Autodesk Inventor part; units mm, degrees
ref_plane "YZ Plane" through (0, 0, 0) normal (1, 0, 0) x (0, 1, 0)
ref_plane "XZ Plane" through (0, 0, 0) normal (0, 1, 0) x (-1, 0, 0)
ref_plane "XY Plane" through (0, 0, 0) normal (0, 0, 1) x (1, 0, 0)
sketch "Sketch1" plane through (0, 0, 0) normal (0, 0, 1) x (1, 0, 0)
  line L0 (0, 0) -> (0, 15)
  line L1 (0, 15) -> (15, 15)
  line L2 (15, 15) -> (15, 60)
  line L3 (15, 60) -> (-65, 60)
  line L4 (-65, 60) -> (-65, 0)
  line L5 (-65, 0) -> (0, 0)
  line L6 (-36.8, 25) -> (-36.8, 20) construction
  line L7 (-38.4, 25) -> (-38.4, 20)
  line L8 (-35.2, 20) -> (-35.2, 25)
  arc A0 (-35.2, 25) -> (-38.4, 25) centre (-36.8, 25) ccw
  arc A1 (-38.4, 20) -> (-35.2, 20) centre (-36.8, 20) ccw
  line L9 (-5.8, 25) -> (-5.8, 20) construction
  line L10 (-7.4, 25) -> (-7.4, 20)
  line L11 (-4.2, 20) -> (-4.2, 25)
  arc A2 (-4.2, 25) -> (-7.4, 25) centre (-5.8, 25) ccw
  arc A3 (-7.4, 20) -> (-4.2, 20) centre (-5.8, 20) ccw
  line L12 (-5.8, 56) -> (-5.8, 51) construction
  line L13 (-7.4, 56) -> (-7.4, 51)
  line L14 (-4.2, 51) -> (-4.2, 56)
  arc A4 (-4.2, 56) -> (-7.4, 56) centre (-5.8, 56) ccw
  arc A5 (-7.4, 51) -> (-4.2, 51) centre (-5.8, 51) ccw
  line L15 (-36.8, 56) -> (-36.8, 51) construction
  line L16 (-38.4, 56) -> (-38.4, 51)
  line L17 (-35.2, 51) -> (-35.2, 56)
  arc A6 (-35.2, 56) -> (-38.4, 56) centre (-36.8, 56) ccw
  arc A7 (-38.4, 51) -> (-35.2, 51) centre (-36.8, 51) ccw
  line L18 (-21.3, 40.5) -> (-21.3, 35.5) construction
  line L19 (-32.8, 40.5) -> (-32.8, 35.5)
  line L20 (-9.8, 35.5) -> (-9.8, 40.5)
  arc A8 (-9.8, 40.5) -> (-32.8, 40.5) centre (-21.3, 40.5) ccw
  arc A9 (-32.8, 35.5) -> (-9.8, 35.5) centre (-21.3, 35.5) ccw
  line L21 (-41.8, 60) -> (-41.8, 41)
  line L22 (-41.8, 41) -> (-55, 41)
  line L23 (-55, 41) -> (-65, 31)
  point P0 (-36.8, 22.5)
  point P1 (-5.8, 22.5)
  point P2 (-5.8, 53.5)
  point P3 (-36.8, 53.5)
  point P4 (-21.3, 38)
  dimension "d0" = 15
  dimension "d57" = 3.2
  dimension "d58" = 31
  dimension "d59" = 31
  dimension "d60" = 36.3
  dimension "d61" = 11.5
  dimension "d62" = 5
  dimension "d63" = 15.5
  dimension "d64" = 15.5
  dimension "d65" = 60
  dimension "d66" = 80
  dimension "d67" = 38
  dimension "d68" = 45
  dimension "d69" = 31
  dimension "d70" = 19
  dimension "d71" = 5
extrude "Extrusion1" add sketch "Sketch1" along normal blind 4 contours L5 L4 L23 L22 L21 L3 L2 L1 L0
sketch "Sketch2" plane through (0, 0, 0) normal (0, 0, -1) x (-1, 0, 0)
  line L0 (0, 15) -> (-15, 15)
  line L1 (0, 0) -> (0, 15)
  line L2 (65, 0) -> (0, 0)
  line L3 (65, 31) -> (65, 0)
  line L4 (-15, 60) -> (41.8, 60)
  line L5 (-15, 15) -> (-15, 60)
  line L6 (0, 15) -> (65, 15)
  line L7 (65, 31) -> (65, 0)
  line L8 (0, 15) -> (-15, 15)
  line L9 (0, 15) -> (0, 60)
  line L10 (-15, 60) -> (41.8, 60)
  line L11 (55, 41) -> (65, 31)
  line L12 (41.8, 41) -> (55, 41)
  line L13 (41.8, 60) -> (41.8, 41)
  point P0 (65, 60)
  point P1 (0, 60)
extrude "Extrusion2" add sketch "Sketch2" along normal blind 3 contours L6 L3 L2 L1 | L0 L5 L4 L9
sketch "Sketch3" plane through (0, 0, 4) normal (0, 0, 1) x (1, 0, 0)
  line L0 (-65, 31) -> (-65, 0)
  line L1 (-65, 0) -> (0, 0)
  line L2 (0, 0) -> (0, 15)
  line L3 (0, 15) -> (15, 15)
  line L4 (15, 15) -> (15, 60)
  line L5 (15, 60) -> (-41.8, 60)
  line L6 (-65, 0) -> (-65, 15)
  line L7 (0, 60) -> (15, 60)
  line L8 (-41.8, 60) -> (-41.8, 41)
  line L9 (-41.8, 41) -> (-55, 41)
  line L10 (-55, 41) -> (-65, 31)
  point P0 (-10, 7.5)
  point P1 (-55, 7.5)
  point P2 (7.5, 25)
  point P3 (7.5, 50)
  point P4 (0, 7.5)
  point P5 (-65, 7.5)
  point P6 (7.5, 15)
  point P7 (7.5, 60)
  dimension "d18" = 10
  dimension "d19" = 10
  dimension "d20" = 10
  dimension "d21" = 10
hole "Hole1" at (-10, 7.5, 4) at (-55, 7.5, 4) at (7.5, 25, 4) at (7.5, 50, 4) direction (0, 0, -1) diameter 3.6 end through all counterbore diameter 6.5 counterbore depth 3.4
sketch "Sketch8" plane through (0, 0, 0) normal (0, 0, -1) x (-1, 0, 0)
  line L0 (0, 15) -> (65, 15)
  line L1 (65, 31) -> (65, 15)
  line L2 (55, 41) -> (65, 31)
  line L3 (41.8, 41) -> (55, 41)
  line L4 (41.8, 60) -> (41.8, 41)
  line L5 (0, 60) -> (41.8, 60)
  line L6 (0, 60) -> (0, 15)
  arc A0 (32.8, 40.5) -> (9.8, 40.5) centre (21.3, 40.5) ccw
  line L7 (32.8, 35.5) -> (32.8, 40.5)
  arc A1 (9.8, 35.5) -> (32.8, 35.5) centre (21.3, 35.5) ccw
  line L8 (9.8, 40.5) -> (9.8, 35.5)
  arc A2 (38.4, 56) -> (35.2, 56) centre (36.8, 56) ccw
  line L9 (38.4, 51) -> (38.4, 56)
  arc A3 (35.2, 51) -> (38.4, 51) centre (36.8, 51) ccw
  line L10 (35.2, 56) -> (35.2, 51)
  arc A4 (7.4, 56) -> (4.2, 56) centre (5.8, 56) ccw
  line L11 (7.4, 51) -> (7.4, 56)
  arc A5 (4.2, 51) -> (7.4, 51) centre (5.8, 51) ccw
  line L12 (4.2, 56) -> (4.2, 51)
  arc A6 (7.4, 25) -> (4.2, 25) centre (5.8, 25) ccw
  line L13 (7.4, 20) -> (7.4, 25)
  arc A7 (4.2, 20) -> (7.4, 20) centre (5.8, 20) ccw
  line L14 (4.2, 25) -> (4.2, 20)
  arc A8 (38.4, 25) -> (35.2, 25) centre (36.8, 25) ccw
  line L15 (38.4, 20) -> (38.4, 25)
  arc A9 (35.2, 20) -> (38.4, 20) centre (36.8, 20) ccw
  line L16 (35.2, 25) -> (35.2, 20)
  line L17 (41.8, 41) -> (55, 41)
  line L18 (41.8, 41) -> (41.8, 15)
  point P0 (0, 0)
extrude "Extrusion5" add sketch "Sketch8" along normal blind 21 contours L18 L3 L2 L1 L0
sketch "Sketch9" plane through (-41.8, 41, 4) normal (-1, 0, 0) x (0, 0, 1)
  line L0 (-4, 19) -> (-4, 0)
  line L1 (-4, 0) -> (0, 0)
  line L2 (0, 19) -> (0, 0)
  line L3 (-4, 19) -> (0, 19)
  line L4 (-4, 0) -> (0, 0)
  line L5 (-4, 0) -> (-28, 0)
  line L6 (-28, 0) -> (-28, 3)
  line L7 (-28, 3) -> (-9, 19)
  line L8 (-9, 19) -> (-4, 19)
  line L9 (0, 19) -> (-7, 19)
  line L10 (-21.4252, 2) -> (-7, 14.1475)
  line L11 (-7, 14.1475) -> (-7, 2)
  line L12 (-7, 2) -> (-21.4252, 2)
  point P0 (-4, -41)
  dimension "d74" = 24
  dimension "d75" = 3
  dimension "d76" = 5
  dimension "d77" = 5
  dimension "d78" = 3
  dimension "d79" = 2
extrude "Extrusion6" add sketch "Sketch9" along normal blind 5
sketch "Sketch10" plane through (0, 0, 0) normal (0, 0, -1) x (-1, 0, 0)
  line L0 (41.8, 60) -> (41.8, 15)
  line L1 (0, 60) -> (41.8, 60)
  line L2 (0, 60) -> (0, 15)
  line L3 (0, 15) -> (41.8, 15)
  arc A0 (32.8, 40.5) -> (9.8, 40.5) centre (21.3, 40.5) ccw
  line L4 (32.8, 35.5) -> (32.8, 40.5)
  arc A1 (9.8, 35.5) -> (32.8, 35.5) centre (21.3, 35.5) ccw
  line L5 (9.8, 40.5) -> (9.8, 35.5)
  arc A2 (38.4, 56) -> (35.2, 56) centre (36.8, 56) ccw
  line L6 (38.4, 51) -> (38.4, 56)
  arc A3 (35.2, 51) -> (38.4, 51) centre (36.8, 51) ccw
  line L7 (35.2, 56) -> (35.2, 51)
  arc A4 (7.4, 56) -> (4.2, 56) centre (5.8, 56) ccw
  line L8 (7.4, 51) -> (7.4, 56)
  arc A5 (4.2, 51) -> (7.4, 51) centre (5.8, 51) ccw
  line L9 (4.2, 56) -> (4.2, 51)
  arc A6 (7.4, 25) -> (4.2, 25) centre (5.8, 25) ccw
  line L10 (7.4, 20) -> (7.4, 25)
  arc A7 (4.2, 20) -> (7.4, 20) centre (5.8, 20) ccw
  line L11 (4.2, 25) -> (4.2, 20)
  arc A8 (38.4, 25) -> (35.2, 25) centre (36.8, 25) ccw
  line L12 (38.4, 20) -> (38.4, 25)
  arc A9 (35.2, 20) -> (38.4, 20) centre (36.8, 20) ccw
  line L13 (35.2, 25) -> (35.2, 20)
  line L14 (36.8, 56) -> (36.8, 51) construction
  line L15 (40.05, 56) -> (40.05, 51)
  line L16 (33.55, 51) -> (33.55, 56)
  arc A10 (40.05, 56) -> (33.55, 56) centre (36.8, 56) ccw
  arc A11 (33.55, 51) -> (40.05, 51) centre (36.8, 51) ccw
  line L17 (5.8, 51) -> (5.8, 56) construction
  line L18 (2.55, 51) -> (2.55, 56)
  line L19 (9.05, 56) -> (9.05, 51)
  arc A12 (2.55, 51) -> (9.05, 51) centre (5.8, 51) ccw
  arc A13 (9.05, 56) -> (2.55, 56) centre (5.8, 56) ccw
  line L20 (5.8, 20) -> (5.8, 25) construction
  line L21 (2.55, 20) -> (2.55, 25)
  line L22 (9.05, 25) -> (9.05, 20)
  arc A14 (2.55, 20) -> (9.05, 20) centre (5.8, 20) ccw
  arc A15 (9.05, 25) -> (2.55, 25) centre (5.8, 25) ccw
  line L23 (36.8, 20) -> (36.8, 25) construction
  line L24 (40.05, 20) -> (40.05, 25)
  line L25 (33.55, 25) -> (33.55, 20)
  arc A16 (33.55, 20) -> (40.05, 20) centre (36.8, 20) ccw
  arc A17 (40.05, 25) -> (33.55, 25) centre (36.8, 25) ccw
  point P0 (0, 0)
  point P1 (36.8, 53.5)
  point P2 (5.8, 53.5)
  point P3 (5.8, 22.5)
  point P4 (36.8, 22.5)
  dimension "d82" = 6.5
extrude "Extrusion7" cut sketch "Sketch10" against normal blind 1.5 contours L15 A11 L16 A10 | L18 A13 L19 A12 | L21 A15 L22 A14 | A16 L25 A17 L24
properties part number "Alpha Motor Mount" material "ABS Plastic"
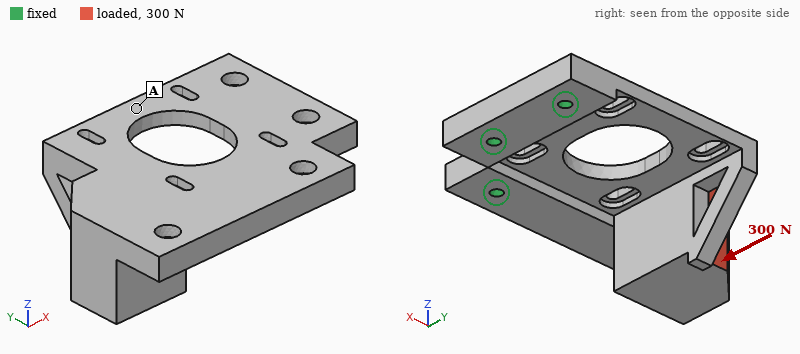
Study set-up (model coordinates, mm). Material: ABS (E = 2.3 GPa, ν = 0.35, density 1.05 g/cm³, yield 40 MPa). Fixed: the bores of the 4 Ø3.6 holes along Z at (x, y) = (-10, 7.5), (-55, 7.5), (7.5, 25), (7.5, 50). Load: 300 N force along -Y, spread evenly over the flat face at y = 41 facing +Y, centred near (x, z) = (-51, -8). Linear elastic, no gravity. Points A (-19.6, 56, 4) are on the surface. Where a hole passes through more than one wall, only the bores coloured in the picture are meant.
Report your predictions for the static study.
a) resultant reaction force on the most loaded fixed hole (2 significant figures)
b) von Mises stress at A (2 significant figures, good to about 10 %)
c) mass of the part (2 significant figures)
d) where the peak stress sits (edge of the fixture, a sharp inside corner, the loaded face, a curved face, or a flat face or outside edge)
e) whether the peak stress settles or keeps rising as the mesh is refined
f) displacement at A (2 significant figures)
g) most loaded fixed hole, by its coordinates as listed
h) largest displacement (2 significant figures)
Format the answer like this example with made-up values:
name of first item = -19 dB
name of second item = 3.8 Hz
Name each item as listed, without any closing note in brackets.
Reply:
resultant reaction force on the most loaded fixed hole = 300 N
von Mises stress at A = 2.4 MPa
mass of the part = 33 g
where the peak stress sits = edge of the fixture
whether the peak stress settles or keeps rising as the mesh is refined = keeps rising
displacement at A = 0.43 mm
most loaded fixed hole, by its coordinates as listed = (-55, 7.5)
largest displacement = 1.1 mm
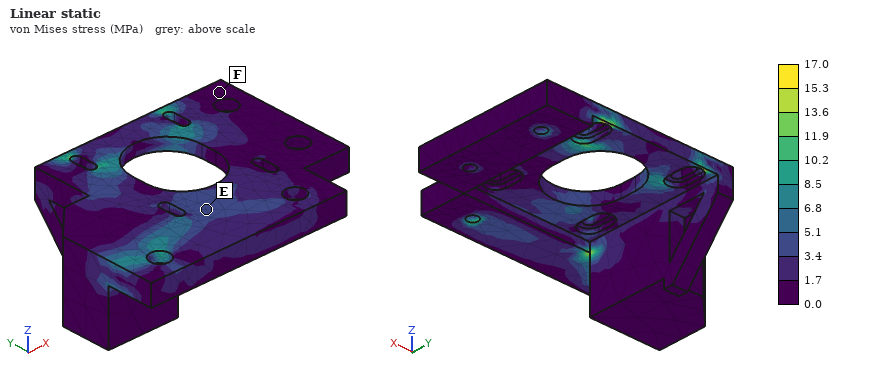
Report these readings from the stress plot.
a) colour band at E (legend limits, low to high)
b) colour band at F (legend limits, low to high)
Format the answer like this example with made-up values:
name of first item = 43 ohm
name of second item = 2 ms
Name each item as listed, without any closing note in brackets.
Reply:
colour band at E = 3.4 to 5.1 MPa
colour band at F = 0.0 to 1.7 MPa
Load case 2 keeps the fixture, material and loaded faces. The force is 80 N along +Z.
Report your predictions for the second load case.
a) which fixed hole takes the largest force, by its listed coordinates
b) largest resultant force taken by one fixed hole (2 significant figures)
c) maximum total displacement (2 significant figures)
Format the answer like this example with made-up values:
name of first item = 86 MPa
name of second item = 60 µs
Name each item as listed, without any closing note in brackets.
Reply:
which fixed hole takes the largest force, by its listed coordinates = (-55, 7.5)
largest resultant force taken by one fixed hole = 84 N
maximum total displacement = 1.1 mm
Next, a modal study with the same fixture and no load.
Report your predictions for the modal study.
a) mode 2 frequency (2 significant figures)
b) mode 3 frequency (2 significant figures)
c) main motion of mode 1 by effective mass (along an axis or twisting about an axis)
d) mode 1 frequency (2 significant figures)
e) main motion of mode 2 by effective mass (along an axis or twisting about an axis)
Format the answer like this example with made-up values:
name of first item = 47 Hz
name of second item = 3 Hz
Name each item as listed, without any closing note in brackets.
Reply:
mode 2 frequency = 1200 Hz
mode 3 frequency = 2400 Hz
main motion of mode 1 by effective mass = along Z
mode 1 frequency = 500 Hz
main motion of mode 2 by effective mass = along X
